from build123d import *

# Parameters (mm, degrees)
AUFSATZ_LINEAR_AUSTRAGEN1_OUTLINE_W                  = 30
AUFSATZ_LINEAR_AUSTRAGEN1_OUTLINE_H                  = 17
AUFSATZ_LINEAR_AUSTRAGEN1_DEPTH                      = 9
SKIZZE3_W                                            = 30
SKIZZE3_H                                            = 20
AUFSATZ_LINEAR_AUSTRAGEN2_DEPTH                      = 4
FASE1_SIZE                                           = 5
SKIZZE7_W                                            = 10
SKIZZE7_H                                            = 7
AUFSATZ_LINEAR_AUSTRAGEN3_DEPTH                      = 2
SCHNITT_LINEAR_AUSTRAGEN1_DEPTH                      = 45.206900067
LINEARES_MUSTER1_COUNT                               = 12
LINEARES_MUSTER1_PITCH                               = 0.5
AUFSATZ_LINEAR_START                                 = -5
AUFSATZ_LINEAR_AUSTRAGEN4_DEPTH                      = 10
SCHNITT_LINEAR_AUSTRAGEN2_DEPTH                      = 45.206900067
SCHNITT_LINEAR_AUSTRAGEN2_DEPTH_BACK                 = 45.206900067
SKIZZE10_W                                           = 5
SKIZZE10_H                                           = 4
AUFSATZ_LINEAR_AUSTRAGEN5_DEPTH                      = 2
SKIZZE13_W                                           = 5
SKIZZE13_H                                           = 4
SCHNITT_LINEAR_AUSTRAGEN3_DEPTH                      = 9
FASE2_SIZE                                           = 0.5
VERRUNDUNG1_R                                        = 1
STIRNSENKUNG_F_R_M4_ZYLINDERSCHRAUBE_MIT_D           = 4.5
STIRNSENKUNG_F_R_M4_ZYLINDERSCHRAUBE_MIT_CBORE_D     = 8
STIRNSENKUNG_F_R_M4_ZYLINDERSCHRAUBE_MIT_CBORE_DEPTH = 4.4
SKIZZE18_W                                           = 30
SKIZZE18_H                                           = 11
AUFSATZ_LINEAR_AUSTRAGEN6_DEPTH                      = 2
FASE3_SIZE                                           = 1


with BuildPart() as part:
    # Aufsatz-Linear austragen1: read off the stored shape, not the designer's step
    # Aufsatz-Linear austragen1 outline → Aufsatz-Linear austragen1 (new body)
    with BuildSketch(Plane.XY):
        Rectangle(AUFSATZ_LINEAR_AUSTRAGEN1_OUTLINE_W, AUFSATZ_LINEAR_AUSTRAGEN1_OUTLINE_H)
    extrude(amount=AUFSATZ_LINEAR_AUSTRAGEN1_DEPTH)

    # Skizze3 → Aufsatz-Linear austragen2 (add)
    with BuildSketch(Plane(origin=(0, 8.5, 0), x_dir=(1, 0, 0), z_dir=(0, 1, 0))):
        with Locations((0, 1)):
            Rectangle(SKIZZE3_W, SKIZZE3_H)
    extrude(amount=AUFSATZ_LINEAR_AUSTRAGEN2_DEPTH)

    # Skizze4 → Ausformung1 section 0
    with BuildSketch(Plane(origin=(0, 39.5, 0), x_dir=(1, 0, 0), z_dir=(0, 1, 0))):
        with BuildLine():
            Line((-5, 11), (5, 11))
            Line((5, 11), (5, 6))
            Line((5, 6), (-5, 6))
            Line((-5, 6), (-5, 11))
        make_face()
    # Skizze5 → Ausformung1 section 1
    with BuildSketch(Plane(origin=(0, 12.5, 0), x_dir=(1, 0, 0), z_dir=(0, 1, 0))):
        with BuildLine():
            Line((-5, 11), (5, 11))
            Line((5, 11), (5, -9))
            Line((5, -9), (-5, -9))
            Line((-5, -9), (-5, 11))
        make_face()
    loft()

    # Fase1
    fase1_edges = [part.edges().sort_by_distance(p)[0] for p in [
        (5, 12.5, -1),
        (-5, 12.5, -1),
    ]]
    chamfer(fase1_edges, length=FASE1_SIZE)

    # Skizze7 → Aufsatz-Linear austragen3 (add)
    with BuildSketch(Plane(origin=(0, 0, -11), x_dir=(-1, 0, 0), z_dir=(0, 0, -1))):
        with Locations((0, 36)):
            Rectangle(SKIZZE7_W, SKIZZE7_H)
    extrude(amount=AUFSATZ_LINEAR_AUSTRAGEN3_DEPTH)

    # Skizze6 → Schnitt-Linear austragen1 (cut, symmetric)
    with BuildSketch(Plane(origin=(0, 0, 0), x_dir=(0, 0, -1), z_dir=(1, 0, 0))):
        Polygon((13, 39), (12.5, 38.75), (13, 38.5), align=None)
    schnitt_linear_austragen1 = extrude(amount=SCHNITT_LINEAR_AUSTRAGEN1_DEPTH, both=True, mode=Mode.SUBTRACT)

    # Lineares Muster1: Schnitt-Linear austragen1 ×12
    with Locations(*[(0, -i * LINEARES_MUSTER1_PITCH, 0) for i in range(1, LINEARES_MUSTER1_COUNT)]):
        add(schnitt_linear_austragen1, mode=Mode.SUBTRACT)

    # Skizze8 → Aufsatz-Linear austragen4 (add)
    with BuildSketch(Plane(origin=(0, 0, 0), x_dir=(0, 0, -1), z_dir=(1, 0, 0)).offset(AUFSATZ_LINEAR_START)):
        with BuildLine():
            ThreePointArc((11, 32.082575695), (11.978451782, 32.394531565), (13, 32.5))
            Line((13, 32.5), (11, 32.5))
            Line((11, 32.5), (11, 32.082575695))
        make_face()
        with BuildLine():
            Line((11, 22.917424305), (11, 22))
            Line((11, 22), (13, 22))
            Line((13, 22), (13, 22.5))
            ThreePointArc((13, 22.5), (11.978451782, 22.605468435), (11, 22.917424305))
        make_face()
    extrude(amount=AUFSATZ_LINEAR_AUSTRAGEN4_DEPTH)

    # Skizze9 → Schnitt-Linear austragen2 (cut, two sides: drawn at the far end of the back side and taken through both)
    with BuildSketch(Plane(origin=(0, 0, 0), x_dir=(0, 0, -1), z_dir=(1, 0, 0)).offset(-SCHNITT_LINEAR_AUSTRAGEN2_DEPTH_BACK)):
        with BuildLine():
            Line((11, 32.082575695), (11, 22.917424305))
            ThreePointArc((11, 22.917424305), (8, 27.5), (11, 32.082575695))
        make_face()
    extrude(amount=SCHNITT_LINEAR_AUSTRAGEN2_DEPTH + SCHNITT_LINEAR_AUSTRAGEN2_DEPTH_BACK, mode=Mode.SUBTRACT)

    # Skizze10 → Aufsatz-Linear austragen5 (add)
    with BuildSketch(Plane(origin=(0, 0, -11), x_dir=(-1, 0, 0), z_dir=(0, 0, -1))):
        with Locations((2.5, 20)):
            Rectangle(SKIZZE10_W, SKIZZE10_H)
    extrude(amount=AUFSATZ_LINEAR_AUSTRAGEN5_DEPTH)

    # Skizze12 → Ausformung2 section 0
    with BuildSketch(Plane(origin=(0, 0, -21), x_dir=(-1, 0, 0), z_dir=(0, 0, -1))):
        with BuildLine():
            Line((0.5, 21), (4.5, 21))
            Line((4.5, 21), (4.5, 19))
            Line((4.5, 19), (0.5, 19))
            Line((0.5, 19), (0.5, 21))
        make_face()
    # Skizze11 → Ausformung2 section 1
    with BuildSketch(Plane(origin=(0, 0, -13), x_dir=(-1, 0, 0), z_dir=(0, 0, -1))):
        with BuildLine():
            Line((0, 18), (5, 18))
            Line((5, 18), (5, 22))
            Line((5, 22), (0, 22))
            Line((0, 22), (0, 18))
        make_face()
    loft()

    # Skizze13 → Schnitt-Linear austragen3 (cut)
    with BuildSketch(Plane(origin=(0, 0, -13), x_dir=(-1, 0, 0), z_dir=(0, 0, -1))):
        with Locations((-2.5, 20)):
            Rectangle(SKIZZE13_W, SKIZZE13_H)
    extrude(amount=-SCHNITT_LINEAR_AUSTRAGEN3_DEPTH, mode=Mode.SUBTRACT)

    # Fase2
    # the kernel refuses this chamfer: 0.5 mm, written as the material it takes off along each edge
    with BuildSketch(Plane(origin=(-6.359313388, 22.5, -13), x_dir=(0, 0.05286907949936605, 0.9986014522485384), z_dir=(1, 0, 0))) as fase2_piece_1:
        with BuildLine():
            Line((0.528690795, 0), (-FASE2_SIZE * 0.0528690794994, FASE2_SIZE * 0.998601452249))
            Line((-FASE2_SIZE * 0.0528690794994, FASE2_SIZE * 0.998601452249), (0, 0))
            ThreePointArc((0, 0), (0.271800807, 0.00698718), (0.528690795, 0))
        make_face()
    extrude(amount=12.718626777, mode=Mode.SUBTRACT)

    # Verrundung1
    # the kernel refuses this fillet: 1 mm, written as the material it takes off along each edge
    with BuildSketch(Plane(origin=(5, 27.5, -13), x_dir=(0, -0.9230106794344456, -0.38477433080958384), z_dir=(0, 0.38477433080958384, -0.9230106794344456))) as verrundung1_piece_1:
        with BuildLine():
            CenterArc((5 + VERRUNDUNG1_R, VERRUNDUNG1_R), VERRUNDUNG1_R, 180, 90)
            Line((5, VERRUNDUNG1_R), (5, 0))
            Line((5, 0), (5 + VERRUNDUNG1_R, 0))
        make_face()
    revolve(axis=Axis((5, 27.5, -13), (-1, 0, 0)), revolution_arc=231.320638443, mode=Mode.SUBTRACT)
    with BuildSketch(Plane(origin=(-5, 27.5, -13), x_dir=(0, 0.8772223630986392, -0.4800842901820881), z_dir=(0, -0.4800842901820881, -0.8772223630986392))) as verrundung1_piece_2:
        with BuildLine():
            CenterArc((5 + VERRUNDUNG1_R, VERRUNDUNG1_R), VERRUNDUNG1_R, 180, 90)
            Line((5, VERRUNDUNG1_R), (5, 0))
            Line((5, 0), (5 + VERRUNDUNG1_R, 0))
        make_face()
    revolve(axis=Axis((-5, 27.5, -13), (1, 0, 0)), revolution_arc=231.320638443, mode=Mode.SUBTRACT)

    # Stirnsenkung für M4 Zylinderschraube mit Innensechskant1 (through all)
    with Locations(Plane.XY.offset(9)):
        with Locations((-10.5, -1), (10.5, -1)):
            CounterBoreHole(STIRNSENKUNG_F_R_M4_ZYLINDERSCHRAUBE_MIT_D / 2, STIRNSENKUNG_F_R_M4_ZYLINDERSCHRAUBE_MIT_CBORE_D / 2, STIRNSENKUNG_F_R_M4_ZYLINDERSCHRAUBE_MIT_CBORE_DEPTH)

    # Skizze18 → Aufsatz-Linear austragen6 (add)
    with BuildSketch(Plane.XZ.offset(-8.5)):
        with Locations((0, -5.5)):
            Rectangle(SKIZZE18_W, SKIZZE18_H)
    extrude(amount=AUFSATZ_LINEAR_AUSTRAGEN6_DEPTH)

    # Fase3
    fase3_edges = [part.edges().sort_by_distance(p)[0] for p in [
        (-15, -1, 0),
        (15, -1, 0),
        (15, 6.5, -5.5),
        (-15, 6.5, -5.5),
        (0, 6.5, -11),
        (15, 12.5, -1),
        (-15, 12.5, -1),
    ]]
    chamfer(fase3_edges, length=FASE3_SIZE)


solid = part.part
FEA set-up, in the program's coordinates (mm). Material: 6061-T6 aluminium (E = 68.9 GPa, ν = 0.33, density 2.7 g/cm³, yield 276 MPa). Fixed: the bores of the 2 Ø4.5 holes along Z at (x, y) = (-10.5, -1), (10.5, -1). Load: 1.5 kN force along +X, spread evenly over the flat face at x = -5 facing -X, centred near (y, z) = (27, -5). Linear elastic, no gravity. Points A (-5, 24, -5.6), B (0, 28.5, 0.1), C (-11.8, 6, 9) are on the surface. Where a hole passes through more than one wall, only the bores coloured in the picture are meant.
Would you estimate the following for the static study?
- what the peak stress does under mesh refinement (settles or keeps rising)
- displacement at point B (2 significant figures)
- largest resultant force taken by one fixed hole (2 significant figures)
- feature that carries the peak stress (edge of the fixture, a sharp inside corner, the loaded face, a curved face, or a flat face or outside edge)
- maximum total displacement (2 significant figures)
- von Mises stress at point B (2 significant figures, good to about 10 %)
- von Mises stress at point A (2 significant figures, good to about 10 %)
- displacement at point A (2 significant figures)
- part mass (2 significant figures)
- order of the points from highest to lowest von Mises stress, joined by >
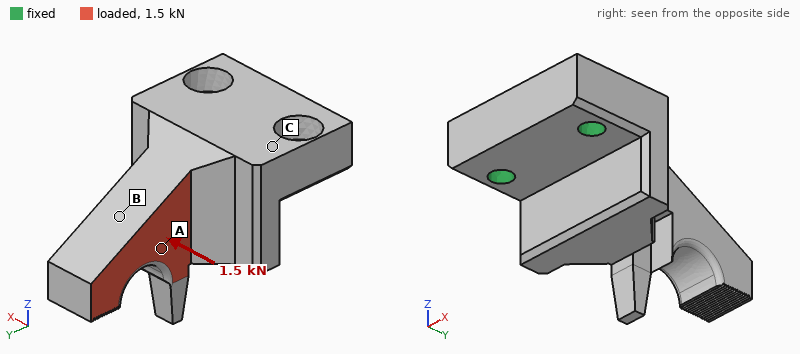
keeps rising
40 µm
2.0 kN
edge of the fixture
98 µm
26 MPa
42 MPa
36 µm
29 g
A > B > C
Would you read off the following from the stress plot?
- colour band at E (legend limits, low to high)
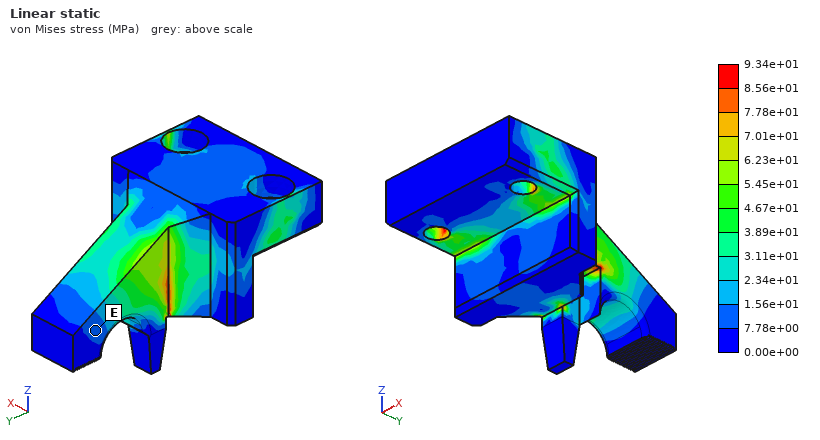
7.78e+00 to 1.56e+01 MPa
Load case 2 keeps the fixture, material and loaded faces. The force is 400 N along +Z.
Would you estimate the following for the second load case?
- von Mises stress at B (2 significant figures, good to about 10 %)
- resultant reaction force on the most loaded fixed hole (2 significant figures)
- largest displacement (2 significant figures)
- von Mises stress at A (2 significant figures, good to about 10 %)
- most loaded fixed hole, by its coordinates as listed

10 MPa
300 N
96 µm
9.2 MPa
(-10.5, -1)
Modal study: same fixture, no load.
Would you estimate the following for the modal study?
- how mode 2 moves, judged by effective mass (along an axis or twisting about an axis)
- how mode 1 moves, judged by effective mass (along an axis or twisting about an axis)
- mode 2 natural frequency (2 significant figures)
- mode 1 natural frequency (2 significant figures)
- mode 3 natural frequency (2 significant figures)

along X
along Z
9500 Hz
4200 Hz
17 kHz
